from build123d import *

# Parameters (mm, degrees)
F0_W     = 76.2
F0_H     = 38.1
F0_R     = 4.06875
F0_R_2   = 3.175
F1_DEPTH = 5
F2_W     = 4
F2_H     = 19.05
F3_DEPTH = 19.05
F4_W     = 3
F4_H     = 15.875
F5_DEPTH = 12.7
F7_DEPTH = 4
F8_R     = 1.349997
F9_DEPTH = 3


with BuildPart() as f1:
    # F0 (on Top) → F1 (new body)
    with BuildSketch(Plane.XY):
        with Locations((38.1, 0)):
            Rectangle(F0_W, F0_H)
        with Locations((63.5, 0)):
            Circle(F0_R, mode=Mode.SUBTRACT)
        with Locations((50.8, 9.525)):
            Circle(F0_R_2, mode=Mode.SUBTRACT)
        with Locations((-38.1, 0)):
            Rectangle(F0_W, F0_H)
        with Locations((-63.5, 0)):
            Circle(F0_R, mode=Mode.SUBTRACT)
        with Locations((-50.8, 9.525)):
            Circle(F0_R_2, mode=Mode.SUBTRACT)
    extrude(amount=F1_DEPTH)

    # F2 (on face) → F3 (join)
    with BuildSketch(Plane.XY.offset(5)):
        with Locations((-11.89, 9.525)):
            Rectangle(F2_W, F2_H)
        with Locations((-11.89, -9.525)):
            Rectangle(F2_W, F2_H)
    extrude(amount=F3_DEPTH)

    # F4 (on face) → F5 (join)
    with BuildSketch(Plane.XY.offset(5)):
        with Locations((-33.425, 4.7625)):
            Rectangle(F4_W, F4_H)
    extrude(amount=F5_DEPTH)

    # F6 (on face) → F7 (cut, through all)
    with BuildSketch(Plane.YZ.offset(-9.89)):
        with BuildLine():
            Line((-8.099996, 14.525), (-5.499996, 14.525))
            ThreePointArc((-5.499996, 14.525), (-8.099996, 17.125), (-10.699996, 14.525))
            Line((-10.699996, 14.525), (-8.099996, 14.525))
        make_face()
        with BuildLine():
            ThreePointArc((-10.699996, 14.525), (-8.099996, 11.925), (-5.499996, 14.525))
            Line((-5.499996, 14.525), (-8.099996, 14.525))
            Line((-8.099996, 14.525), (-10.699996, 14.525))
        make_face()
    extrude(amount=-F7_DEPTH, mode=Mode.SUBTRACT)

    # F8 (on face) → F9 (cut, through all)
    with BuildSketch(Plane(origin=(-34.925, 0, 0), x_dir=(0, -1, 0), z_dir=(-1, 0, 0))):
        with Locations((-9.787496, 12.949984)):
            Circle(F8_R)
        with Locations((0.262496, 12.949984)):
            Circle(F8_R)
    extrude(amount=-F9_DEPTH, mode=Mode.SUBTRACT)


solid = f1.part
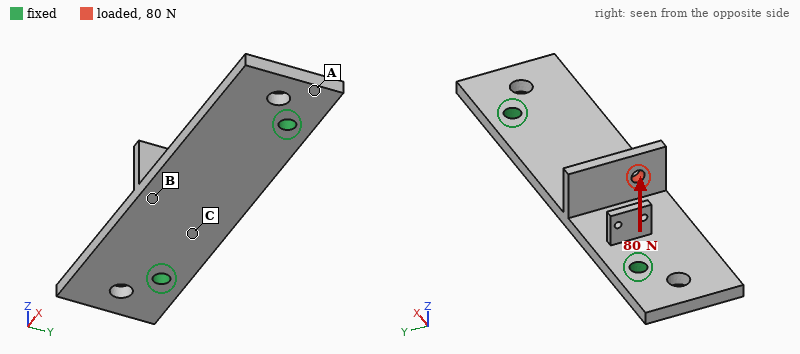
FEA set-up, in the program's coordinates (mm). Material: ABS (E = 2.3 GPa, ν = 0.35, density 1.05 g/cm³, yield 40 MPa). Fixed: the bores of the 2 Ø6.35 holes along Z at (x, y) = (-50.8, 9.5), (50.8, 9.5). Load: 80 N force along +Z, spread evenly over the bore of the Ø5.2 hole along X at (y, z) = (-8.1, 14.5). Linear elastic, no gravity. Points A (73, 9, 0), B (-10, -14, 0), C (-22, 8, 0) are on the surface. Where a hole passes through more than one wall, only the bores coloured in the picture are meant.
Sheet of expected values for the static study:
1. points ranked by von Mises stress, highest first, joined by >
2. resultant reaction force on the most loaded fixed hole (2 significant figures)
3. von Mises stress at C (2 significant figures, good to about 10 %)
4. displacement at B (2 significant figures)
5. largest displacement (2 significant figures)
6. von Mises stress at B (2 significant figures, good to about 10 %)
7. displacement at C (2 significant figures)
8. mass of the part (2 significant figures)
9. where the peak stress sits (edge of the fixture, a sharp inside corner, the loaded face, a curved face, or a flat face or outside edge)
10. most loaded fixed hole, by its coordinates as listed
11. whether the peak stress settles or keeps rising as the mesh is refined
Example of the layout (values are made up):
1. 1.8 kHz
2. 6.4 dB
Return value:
1. B > C > A
2. 53 N
3. 2.7 MPa
4. 0.75 mm
5. 0.91 mm
6. 6.2 MPa
7. 0.30 mm
8. 33 g
9. edge of the fixture
10. (-50.8, 9.5)
11. keeps rising
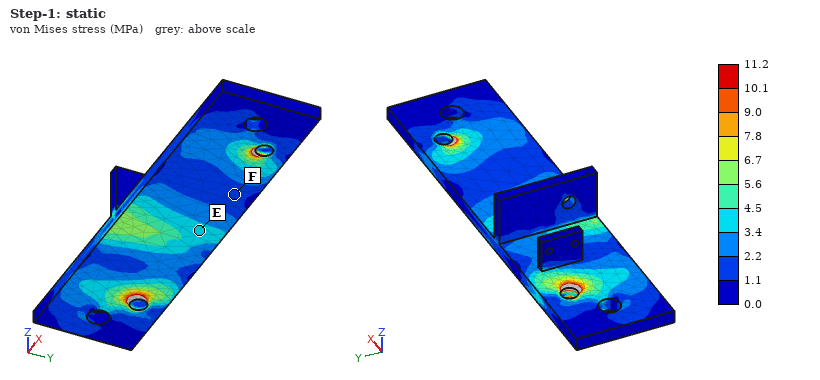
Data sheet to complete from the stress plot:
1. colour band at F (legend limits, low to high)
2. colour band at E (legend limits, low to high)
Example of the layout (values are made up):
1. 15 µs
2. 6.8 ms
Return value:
1. 1.1 to 2.2 MPa
2. 3.4 to 4.5 MPa
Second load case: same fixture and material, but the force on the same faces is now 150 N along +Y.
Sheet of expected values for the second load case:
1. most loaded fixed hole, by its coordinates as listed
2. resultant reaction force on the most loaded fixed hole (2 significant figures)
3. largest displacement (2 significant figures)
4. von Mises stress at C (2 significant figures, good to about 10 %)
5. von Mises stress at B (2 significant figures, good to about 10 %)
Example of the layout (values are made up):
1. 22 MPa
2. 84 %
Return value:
1. (-50.8, 9.5)
2. 110 N
3. 1.00 mm
4. 3.8 MPa
5. 6.0 MPa
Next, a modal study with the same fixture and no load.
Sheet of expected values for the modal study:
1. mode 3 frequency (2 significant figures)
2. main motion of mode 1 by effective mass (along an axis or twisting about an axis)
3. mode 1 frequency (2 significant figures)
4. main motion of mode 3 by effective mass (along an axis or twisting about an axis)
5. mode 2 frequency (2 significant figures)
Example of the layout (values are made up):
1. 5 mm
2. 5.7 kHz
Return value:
1. 1200 Hz
2. along Z
3. 560 Hz
4. twisting about Y
5. 870 Hz
